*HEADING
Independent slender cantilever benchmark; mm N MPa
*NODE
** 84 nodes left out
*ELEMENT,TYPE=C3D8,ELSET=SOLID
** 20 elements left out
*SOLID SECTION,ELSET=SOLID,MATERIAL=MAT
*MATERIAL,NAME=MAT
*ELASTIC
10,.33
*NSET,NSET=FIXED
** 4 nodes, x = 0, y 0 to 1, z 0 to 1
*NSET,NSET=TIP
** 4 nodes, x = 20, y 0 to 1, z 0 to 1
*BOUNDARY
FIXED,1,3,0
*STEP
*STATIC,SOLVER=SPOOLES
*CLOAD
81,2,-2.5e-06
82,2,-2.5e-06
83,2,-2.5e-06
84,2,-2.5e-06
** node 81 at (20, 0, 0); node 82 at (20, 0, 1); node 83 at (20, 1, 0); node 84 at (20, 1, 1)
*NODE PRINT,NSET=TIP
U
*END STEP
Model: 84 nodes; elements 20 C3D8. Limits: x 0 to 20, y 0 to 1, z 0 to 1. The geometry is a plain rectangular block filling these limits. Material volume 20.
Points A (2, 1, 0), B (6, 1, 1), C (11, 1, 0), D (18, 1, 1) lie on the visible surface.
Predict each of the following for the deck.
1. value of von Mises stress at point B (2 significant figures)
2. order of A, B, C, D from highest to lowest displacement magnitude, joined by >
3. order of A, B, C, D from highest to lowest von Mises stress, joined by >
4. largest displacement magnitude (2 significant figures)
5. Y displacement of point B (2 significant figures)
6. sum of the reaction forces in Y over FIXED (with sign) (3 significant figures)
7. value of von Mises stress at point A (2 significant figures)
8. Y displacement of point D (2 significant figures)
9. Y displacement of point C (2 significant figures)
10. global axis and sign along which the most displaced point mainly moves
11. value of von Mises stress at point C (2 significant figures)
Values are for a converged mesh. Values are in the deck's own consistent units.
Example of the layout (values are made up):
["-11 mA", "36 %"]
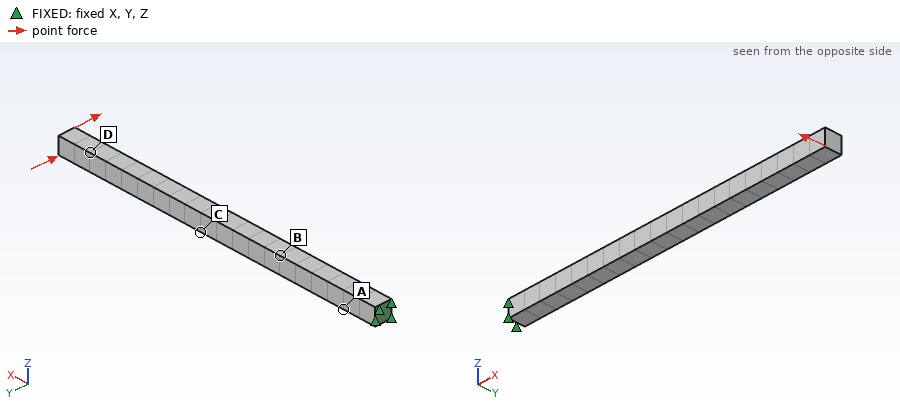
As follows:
["8.4e-04", "D > C > B > A", "A > B > C > D", "0.032", "-0.0038", "1.00e-05", "0.0011", "-0.027", "-0.012", "-Y", "5.4e-04"]
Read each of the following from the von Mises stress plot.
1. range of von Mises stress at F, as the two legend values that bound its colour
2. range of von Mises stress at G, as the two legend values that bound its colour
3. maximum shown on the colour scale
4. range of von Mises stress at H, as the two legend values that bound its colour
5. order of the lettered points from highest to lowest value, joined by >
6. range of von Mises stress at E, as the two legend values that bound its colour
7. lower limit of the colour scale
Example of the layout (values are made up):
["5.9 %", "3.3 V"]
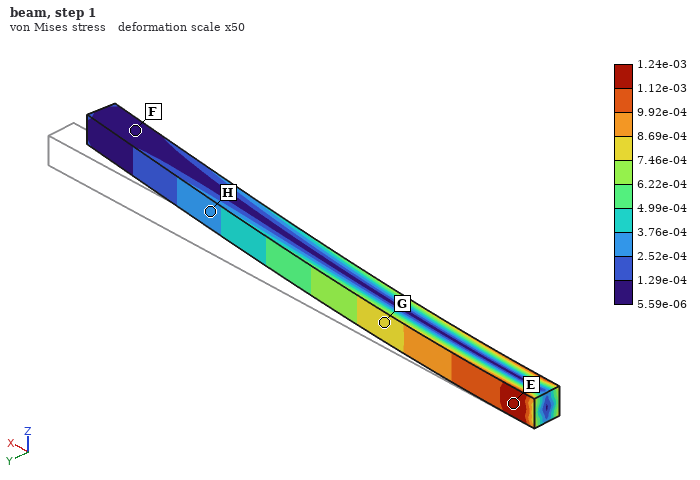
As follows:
["5.59e-06 to 1.29e-04", "7.46e-04 to 8.69e-04", "1.24e-03", "2.52e-04 to 3.76e-04", "E > G > H > F", "1.12e-03 to 1.24e-03", "5.59e-06"]
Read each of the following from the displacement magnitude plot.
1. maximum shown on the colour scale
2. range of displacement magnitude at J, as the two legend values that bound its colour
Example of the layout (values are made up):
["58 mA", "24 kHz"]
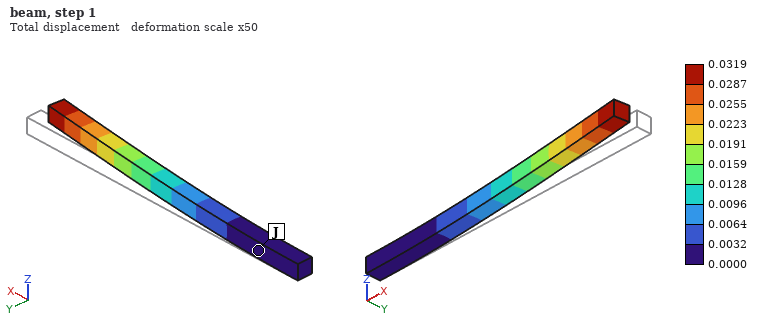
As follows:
["0.0319", "0.0000 to 0.0032"]
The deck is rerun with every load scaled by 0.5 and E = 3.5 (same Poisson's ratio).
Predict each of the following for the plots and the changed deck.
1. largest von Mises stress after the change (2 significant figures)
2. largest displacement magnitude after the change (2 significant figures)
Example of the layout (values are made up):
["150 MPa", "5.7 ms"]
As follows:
["6.2e-04", "0.046"]
